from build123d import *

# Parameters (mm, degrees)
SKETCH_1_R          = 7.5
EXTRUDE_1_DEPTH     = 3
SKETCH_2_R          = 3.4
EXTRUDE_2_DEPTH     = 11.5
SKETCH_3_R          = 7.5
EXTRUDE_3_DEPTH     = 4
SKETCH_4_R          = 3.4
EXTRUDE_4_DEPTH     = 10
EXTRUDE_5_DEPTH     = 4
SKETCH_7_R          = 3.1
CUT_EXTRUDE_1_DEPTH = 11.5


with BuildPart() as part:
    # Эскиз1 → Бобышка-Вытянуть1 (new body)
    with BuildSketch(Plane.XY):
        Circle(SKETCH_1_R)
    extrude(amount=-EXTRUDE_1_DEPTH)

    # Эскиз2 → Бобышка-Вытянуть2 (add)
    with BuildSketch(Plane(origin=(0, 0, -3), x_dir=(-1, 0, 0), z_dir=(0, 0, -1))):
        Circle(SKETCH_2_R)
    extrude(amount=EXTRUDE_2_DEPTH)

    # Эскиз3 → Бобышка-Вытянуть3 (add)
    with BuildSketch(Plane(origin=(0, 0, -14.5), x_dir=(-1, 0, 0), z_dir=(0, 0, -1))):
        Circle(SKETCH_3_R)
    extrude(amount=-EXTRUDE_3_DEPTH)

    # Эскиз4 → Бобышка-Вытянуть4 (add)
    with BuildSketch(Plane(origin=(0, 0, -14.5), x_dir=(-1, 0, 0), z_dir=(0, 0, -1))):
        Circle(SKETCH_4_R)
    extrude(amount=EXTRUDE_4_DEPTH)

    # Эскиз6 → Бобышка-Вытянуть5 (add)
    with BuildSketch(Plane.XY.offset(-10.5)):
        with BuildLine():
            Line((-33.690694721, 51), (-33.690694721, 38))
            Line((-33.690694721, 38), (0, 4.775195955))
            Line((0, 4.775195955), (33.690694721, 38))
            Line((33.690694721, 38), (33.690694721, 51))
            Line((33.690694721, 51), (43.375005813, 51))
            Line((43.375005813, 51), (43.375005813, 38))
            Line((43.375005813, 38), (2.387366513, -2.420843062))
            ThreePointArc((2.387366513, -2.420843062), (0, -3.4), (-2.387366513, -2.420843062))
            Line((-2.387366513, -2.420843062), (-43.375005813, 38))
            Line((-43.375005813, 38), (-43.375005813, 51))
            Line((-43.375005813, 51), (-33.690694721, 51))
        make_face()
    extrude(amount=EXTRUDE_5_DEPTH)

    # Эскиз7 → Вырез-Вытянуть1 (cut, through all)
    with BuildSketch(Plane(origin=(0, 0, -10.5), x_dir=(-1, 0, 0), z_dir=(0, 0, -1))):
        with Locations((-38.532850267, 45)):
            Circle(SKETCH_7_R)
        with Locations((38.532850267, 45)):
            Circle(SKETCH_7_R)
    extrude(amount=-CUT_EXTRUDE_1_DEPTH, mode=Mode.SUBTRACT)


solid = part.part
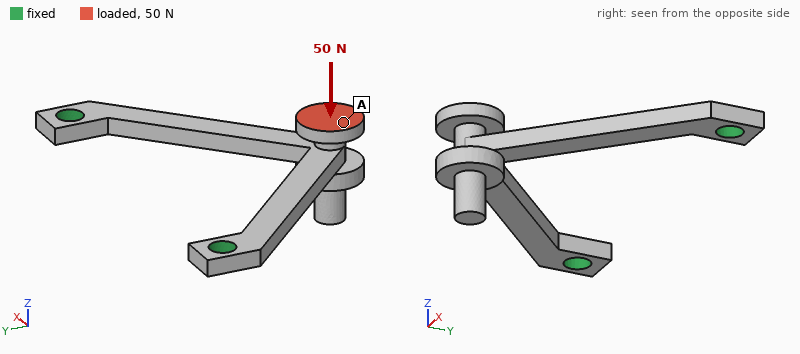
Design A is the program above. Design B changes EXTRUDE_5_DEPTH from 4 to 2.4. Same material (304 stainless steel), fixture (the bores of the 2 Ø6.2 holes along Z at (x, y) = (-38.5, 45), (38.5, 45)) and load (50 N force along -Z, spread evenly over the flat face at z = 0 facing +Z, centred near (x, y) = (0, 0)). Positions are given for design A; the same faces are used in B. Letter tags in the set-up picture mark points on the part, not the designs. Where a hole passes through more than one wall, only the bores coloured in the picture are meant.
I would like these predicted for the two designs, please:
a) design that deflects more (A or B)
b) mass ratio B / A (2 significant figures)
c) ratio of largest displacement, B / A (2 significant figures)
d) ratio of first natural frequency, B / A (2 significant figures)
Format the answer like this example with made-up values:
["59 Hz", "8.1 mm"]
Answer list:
["B", "0.74", "4.2", "0.51"]
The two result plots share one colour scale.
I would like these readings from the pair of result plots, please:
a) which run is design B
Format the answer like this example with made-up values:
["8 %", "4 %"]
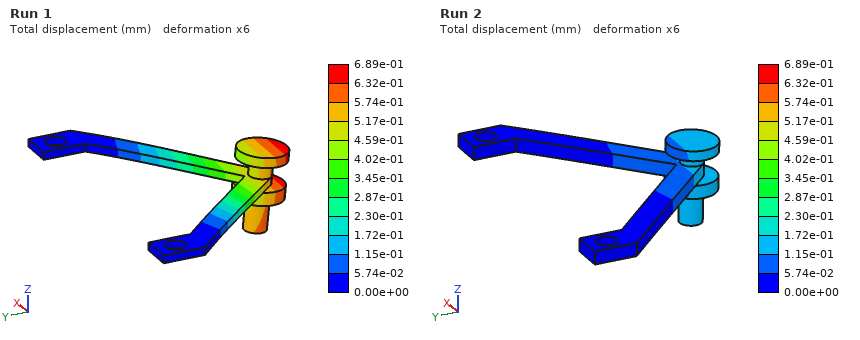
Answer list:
["Run 1"]
